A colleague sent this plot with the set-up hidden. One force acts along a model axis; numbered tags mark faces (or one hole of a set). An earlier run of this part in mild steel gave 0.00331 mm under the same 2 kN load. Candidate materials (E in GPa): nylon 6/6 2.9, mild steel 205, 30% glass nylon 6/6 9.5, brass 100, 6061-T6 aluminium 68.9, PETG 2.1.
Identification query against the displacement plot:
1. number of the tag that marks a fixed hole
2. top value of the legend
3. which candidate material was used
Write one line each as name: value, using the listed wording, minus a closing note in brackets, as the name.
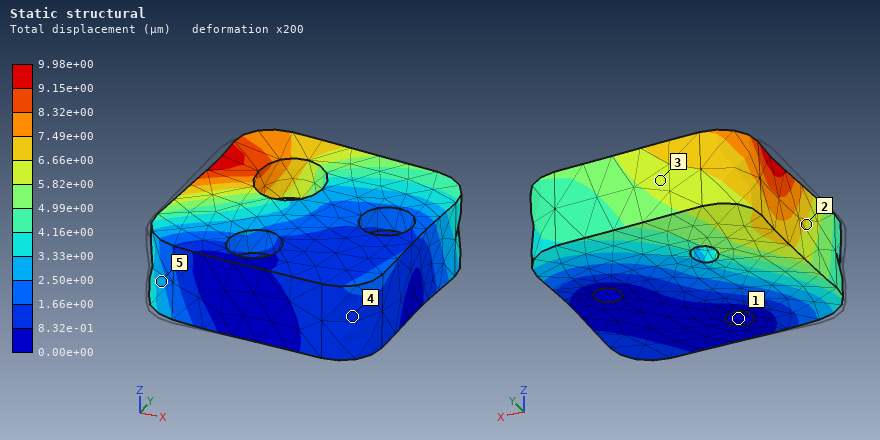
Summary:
number of the tag that marks a fixed hole: 1
top value of the legend: 9.98e+00 µm
which candidate material was used: 6061-T6 aluminium
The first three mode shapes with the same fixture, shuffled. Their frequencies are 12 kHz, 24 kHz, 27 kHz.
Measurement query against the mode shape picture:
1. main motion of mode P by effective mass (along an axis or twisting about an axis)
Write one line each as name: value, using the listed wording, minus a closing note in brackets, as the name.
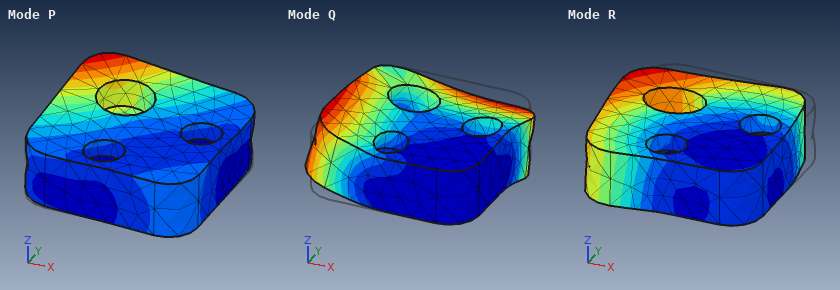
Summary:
main motion of mode P by effective mass: along Z
